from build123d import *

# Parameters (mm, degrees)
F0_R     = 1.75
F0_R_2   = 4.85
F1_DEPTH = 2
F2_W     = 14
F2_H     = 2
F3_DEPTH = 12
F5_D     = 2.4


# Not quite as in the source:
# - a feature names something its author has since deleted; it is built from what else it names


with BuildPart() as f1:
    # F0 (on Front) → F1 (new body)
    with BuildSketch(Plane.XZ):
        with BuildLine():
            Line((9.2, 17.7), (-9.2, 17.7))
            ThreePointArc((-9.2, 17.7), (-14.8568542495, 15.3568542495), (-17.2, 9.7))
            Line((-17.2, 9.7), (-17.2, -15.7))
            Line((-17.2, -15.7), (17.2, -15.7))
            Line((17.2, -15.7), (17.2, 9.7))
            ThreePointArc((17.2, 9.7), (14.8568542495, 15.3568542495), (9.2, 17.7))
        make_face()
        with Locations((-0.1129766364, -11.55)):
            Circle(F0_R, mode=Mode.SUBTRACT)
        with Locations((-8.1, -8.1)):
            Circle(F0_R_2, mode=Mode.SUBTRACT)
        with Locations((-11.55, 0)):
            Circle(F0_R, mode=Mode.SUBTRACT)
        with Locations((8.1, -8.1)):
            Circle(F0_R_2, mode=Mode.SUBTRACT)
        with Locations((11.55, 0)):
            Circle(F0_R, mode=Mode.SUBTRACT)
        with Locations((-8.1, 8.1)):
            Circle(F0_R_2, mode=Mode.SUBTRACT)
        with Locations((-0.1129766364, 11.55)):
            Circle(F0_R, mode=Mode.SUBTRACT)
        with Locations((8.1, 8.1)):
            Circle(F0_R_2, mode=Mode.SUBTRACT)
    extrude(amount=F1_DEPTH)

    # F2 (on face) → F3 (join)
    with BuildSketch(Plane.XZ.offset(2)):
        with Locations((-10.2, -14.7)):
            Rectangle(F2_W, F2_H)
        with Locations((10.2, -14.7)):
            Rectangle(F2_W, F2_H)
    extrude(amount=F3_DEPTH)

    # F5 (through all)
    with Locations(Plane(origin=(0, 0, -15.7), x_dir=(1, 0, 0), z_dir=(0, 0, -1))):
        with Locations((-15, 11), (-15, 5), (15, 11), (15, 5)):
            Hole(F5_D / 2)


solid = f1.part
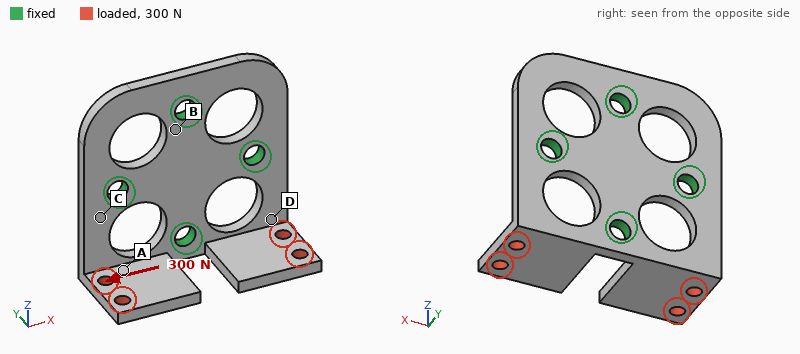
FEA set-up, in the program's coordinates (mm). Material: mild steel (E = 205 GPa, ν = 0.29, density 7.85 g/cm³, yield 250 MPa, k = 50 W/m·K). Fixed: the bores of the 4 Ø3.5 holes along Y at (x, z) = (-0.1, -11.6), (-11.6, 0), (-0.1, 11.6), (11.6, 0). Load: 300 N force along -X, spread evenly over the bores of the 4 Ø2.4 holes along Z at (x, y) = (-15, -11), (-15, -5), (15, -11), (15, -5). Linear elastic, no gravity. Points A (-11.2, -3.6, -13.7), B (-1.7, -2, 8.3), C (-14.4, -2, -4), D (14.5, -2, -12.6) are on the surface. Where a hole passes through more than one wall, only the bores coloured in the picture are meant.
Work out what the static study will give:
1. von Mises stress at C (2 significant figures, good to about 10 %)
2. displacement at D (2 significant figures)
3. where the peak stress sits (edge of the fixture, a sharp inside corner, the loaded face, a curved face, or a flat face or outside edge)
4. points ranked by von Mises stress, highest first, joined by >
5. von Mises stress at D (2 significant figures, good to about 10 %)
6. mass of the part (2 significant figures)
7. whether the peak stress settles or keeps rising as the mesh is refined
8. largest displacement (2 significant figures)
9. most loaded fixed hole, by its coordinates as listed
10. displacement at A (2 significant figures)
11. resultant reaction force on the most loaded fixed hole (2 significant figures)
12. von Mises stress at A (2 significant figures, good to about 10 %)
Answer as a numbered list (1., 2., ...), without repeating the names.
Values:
1. 79 MPa
2. 24 µm
3. a sharp inside corner
4. C > D > A > B
5. 45 MPa
6. 17 g
7. keeps rising
8. 57 µm
9. (-0.1, -11.6)
10. 21 µm
11. 280 N
12. 28 MPa
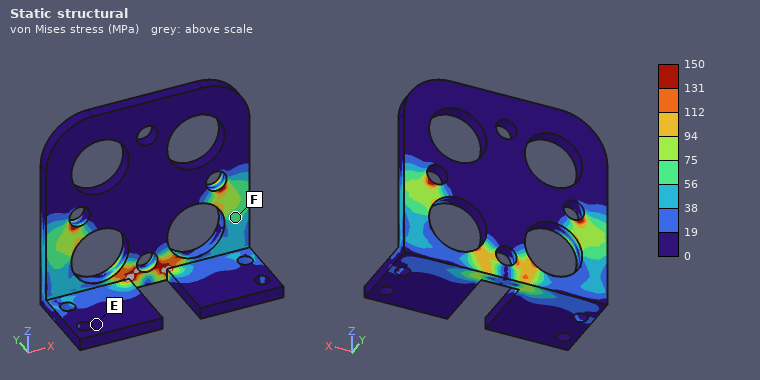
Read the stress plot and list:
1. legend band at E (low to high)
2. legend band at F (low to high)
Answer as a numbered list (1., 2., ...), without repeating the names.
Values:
1. 0 to 19 MPa
2. 56 to 75 MPa
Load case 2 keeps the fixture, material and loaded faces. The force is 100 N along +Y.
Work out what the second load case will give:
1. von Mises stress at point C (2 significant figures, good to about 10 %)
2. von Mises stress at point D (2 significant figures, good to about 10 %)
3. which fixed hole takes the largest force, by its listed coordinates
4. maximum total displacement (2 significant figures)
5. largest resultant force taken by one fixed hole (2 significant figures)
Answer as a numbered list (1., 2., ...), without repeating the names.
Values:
1. 48 MPa
2. 24 MPa
3. (-0.1, -11.6)
4. 35 µm
5. 51 N
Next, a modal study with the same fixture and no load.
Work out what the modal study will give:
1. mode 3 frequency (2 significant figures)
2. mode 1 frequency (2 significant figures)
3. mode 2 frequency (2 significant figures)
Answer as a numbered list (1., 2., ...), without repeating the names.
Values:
1. 7500 Hz
2. 4300 Hz
3. 4400 Hz
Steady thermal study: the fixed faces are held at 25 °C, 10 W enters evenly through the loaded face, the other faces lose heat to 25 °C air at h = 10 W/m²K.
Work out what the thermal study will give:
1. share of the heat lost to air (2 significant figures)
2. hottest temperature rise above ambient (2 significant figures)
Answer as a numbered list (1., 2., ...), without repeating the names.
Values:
1. 6.0 %
2. 80 K
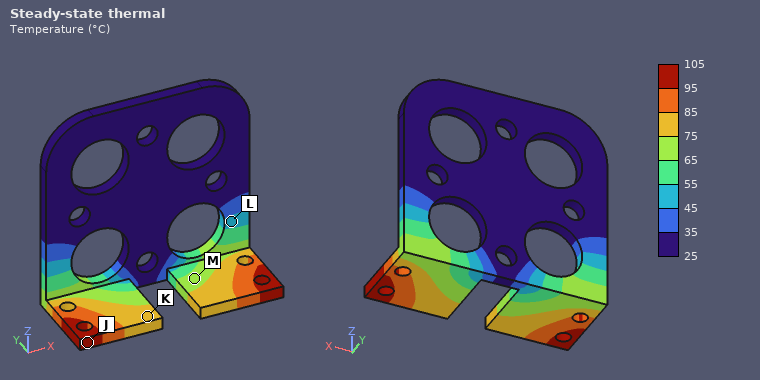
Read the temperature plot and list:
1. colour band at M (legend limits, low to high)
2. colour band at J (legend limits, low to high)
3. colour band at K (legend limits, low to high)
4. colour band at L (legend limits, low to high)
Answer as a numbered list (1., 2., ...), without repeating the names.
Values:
1. 65 to 75 °C
2. 95 to 105 °C
3. 75 to 85 °C
4. 45 to 55 °C
